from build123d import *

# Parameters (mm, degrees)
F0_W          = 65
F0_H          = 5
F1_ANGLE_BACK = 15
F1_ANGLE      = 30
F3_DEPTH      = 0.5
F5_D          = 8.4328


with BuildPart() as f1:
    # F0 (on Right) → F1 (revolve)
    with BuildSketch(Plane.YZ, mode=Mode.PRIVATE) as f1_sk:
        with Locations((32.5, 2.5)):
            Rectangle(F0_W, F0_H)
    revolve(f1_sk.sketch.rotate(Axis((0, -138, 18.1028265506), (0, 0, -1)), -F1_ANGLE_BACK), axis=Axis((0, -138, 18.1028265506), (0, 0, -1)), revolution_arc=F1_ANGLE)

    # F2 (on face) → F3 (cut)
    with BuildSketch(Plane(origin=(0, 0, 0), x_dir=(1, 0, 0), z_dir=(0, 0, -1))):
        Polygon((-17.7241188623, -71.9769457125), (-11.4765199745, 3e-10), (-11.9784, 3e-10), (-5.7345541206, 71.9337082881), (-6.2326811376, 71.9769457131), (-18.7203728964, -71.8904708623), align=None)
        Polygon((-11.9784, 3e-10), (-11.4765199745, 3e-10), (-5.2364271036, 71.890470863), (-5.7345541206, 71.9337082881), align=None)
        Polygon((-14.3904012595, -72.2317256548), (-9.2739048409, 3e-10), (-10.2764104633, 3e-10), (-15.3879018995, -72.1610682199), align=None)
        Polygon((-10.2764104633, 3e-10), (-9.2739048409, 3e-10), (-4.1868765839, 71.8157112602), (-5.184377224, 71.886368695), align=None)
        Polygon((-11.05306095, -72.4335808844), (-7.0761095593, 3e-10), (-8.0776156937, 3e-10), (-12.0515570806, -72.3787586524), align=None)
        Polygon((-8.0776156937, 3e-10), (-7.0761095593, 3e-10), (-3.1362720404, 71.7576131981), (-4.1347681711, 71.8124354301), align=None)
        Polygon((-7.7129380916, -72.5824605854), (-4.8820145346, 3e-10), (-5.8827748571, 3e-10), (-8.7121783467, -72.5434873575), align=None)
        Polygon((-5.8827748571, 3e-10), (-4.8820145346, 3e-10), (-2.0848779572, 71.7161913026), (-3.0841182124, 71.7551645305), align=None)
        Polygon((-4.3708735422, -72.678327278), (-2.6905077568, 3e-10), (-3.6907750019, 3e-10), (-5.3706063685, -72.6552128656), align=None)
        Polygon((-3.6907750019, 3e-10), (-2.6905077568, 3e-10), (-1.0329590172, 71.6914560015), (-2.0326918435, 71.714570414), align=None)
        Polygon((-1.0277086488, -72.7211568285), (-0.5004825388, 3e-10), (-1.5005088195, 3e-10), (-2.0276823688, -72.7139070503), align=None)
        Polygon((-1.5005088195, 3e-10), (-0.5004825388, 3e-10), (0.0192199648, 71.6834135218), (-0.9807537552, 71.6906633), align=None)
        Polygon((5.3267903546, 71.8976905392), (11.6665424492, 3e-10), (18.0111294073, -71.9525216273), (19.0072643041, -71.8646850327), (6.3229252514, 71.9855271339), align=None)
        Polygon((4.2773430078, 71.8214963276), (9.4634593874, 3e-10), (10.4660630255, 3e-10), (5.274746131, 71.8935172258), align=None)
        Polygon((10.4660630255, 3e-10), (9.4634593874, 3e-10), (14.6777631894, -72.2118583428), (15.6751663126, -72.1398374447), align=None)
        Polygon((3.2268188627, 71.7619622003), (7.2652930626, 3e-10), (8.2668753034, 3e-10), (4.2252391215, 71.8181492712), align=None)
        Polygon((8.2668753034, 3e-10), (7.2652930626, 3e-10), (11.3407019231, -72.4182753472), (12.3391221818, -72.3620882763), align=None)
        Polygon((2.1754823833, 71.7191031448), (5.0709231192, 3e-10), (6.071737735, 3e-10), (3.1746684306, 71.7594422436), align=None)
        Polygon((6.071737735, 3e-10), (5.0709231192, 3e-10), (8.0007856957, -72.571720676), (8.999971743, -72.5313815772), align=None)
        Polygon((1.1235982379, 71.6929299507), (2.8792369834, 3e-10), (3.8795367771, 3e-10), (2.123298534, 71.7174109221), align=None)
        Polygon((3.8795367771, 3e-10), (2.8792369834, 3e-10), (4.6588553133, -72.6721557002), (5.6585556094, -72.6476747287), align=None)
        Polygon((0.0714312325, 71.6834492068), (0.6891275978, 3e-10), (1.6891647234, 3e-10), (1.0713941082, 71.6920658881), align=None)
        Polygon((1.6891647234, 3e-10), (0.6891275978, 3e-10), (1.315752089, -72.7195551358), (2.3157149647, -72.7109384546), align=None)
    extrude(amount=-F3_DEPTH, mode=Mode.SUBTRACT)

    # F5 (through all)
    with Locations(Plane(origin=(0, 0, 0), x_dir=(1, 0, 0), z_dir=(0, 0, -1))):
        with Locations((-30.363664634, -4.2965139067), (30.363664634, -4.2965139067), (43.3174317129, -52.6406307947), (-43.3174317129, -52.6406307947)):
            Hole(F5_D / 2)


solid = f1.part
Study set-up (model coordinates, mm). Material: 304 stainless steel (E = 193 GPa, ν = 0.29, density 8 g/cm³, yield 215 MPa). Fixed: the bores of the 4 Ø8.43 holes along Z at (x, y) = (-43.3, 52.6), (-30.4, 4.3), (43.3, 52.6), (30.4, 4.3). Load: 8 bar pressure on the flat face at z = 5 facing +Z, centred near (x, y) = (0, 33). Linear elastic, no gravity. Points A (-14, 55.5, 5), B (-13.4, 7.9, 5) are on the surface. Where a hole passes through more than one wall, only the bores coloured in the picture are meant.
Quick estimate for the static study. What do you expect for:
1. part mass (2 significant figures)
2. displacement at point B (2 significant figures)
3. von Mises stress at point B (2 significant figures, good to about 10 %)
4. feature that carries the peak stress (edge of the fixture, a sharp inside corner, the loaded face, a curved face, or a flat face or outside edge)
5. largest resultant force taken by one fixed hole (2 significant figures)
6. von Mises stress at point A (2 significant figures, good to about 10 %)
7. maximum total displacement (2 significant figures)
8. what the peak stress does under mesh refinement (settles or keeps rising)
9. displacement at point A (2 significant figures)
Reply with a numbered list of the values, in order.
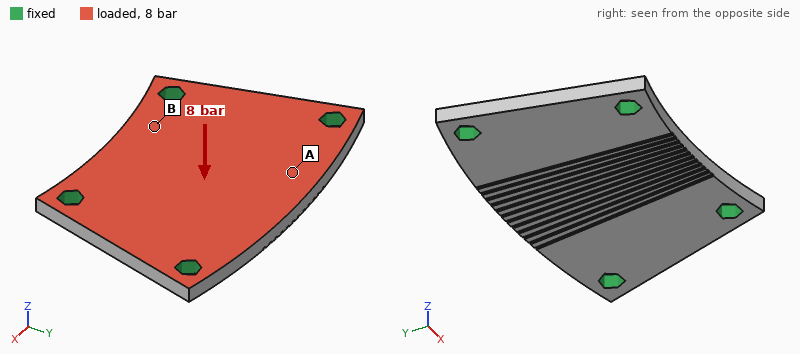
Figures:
1. 220 g
2. 12 µm
3. 19 MPa
4. edge of the fixture
5. 1.2 kN
6. 39 MPa
7. 62 µm
8. keeps rising
9. 44 µm
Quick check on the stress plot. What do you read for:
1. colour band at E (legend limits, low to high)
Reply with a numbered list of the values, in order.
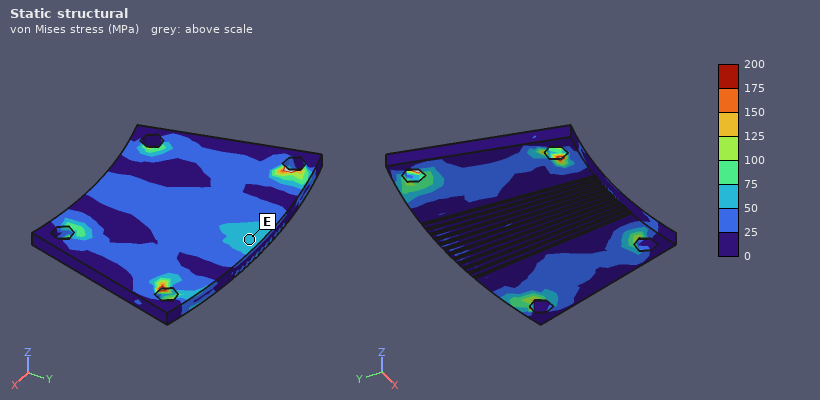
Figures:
1. 50 to 75 MPa
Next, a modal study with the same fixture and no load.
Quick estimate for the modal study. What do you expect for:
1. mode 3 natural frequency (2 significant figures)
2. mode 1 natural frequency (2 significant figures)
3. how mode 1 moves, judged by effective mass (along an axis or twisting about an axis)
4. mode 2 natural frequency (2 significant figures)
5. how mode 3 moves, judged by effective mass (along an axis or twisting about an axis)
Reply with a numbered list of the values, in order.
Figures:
1. 9400 Hz
2. 3800 Hz
3. along Z
4. 6800 Hz
5. twisting about Y
